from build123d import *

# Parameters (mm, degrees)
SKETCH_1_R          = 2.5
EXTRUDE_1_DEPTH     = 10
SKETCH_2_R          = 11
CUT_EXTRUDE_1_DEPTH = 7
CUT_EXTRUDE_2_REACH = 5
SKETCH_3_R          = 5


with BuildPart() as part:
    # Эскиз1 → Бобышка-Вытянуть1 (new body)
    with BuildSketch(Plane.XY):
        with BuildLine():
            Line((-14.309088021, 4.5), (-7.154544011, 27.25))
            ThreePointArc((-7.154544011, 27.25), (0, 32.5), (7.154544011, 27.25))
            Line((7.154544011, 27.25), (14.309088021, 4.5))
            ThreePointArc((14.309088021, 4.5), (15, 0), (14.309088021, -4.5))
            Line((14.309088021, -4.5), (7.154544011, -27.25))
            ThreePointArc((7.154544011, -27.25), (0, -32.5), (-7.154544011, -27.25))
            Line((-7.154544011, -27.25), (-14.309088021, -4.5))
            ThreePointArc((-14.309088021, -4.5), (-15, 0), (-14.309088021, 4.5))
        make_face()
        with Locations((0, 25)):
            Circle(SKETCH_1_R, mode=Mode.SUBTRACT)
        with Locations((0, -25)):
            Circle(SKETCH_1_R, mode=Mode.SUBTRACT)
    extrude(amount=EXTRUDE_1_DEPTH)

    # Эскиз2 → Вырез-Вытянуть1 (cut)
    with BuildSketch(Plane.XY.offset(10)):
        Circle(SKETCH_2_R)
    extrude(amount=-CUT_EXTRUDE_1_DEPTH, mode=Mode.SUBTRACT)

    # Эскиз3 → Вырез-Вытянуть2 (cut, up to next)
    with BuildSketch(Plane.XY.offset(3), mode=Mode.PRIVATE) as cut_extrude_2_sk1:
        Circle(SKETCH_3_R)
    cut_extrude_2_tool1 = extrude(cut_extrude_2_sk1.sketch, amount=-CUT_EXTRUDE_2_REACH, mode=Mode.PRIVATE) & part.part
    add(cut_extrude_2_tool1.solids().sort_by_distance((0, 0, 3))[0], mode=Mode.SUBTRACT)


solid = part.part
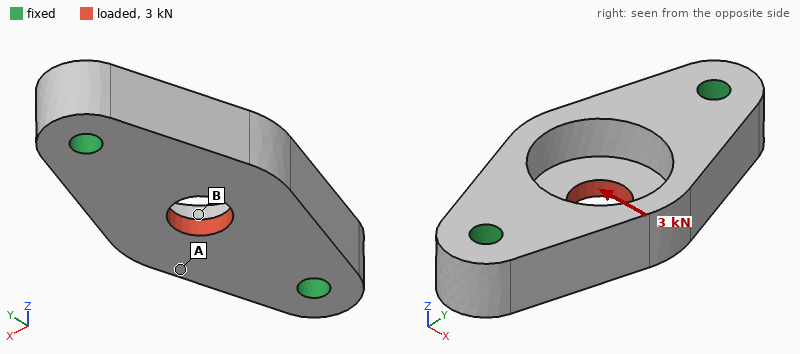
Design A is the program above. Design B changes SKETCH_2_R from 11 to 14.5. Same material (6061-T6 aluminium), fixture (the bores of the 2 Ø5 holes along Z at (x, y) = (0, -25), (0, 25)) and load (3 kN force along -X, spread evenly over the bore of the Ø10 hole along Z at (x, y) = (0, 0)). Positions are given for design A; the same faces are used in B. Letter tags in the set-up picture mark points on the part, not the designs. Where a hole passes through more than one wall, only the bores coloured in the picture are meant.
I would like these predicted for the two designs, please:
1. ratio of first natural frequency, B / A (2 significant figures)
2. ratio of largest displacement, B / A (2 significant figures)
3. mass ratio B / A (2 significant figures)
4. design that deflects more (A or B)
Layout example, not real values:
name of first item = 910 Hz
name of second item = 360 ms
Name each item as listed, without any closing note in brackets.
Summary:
ratio of first natural frequency, B / A = 1.0
ratio of largest displacement, B / A = 1.3
mass ratio B / A = 0.81
design that deflects more = B
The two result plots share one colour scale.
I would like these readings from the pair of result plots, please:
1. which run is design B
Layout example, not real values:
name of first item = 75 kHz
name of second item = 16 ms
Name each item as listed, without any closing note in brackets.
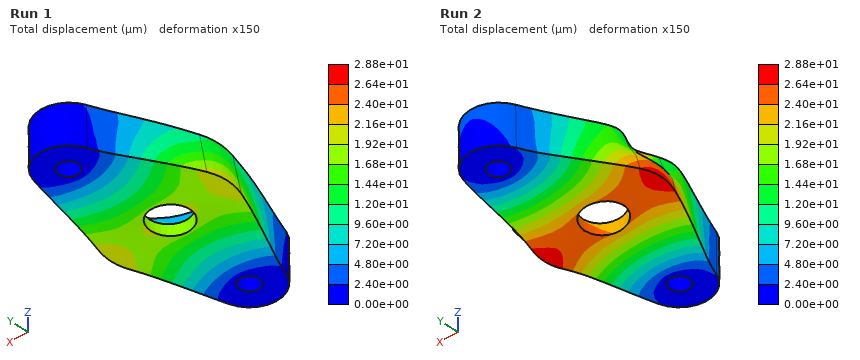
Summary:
which run is design B = Run 2
